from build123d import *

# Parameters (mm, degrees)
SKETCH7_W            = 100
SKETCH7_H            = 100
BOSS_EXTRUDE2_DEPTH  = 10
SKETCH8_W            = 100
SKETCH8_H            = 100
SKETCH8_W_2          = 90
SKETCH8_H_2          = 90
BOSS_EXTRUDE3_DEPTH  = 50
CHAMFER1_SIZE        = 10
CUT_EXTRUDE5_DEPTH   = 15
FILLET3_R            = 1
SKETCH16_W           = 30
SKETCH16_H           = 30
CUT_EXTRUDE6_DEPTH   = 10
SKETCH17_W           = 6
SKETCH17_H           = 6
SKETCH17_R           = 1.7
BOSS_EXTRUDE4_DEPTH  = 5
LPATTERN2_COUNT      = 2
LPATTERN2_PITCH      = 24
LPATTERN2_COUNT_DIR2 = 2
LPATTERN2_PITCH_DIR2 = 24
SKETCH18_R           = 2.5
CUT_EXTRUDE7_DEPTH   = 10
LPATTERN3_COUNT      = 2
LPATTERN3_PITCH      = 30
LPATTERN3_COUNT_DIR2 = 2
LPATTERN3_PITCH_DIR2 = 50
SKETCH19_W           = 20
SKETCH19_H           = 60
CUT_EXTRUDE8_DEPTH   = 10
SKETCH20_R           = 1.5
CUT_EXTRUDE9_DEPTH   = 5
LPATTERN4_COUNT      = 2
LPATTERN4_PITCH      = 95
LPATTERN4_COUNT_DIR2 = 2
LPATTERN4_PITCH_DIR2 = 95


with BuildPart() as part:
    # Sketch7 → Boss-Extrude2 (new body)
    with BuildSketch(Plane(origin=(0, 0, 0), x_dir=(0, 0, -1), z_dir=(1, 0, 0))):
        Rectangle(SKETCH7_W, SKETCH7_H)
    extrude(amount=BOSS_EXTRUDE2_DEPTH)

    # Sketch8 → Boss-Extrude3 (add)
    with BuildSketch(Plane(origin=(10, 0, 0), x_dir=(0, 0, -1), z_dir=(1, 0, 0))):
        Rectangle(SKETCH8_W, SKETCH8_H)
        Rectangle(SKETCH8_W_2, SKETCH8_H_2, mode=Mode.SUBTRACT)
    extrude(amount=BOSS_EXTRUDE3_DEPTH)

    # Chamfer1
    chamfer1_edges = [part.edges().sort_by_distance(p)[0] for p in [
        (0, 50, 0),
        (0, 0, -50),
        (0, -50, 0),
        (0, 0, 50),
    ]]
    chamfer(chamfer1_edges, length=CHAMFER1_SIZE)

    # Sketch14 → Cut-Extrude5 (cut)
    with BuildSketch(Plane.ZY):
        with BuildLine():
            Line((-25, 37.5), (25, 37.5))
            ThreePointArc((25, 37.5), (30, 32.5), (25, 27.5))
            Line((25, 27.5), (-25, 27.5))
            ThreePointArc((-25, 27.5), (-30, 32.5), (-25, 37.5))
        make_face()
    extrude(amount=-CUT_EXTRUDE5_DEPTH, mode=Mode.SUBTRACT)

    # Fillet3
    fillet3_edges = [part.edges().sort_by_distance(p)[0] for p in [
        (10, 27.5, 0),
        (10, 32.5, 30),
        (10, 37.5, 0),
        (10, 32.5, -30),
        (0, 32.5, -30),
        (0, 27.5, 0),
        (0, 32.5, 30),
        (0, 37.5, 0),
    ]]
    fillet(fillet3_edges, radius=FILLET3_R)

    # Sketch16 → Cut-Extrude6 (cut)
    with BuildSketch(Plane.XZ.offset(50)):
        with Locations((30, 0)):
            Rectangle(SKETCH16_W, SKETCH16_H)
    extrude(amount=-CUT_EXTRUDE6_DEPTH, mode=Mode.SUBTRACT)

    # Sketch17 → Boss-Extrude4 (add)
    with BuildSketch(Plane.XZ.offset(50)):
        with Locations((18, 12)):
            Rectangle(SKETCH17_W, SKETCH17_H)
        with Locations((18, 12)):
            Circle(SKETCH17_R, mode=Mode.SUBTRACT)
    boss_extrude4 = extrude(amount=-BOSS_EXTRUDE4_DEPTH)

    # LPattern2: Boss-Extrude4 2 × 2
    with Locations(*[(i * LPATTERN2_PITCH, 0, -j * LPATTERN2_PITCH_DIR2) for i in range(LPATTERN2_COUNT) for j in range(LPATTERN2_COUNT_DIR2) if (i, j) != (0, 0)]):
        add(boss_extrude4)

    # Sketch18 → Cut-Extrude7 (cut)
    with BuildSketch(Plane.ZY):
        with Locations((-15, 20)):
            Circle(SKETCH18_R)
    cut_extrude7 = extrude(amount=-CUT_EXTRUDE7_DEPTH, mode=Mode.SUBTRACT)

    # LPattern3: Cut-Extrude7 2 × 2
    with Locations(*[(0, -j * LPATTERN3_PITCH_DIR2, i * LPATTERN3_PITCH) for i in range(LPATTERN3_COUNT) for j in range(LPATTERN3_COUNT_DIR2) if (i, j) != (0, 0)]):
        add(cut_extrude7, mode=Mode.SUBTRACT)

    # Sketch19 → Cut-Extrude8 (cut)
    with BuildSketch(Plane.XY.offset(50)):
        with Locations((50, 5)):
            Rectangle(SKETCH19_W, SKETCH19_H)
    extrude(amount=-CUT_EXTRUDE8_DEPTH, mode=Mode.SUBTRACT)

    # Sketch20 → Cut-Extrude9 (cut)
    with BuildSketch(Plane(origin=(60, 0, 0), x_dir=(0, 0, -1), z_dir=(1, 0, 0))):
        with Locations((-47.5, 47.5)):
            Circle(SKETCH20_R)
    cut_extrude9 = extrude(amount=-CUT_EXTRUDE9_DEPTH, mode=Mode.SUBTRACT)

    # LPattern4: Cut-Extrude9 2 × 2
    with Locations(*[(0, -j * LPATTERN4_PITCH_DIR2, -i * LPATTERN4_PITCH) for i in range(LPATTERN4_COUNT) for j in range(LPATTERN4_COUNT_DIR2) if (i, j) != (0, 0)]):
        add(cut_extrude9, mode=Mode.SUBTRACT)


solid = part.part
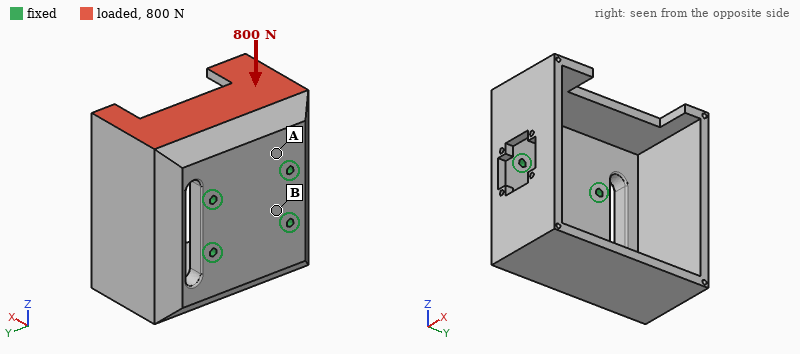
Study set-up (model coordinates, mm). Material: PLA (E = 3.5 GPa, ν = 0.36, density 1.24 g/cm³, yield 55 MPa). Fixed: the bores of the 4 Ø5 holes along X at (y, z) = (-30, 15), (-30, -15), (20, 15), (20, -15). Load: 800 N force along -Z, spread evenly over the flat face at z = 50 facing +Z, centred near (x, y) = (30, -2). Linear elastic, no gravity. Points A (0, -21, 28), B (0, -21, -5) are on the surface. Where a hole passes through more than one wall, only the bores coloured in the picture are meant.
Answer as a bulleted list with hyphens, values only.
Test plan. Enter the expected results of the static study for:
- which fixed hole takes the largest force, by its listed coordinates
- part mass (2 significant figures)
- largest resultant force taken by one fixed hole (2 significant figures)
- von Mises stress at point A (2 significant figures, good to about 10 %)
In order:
- (20, 15)
- 200 g
- 360 N
- 3.1 MPa
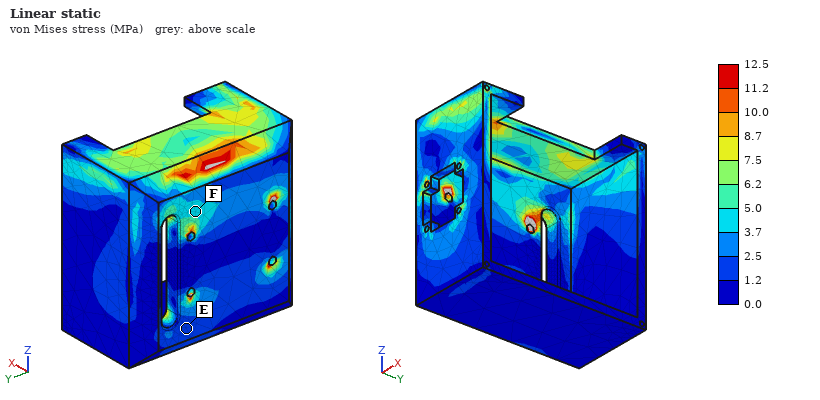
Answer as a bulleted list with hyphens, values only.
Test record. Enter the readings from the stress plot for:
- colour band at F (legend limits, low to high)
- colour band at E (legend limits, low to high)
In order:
- 3.7 to 5.0 MPa
- 1.2 to 2.5 MPa
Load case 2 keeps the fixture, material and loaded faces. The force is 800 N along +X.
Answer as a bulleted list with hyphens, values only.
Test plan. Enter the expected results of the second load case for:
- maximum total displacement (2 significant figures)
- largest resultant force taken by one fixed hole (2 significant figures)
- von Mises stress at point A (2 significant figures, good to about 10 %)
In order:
- 0.71 mm
- 640 N
- 5.8 MPa
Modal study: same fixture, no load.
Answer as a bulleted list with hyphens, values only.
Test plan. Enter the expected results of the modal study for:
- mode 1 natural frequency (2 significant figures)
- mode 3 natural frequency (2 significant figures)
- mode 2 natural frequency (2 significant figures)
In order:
- 590 Hz
- 760 Hz
- 660 Hz
